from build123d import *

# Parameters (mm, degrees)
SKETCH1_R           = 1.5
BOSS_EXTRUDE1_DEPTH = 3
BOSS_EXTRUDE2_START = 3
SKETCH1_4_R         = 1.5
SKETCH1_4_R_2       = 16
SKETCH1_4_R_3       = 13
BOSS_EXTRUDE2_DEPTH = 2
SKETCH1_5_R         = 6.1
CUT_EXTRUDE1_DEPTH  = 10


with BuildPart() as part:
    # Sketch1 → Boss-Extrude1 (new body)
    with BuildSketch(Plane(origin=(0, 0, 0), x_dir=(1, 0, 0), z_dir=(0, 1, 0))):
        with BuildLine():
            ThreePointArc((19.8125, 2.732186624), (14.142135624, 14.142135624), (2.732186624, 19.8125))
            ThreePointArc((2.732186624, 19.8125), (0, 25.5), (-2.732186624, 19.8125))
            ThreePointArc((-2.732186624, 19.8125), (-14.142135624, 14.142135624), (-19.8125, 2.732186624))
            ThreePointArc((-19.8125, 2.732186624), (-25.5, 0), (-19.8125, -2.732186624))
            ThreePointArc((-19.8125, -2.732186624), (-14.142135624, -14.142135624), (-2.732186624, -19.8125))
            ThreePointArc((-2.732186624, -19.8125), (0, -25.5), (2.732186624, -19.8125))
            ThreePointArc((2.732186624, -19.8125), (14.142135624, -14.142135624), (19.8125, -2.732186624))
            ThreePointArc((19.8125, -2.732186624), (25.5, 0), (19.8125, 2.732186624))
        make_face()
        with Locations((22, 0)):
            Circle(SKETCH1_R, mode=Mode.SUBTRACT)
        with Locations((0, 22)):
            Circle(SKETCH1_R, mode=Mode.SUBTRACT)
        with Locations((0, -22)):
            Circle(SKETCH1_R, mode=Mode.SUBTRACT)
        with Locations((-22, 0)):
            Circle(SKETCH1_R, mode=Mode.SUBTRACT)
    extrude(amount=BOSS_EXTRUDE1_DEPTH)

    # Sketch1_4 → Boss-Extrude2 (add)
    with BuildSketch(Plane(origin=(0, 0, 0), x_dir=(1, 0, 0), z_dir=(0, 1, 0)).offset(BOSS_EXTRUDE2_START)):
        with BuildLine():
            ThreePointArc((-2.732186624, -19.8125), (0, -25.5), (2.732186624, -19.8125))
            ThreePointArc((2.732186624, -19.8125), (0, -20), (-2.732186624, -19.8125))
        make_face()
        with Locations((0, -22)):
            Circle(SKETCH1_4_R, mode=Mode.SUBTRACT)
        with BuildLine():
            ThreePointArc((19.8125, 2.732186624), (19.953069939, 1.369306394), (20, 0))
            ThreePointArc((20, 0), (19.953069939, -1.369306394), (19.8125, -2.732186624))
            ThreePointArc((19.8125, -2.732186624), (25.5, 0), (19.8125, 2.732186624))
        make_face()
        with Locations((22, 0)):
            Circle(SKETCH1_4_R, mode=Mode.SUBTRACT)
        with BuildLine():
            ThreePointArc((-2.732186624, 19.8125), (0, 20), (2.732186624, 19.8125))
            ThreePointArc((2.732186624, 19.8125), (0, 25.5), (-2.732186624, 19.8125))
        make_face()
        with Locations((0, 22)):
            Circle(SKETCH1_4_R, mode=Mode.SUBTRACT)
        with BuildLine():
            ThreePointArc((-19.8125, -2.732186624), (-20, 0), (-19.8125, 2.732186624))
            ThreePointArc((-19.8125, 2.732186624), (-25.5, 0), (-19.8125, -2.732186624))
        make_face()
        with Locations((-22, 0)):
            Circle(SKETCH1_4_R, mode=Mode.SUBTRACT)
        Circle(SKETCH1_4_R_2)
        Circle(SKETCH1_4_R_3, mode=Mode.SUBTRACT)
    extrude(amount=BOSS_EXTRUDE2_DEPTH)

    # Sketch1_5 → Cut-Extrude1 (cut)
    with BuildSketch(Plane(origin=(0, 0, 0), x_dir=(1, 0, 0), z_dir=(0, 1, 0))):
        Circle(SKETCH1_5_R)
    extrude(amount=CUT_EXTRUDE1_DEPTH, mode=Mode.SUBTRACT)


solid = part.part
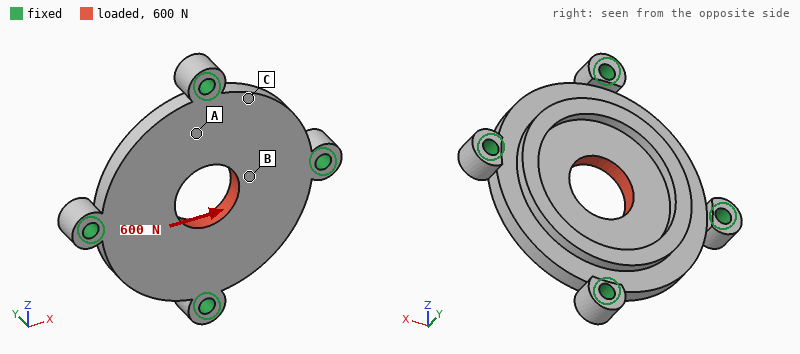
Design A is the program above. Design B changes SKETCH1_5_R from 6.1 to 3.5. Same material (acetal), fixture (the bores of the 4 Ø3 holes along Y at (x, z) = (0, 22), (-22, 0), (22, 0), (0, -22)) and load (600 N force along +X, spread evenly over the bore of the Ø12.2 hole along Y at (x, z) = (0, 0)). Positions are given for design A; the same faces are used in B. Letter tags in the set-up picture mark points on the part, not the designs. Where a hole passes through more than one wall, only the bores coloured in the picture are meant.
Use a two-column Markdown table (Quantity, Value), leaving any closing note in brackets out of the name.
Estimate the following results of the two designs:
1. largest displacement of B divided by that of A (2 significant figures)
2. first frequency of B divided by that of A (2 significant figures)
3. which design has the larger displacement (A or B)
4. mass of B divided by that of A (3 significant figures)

| Quantity | Value |
|---|---|
| largest displacement of B divided by that of A | 1.2 |
| first frequency of B divided by that of A | 0.95 |
| which design has the larger displacement | B |
| mass of B divided by that of A | 1.05 |
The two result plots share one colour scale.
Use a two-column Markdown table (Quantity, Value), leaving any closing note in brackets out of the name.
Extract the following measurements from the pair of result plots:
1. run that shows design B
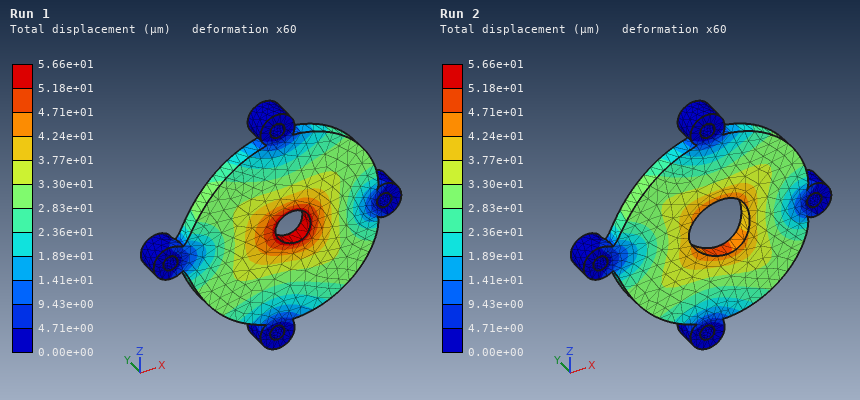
| Quantity | Value |
|---|---|
| run that shows design B | Run 1 |
